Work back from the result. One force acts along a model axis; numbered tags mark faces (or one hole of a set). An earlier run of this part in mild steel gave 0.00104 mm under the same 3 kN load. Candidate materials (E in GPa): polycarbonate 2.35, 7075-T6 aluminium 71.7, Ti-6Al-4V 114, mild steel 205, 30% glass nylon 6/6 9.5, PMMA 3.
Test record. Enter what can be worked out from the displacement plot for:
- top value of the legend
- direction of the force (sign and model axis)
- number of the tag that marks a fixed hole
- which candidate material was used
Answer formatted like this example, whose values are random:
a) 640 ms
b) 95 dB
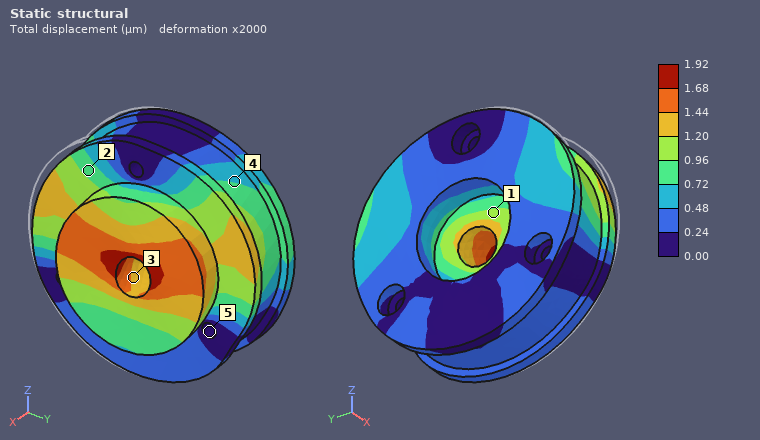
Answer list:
a) 1.92 µm
b) +Y
c) 5
d) Ti-6Al-4V
